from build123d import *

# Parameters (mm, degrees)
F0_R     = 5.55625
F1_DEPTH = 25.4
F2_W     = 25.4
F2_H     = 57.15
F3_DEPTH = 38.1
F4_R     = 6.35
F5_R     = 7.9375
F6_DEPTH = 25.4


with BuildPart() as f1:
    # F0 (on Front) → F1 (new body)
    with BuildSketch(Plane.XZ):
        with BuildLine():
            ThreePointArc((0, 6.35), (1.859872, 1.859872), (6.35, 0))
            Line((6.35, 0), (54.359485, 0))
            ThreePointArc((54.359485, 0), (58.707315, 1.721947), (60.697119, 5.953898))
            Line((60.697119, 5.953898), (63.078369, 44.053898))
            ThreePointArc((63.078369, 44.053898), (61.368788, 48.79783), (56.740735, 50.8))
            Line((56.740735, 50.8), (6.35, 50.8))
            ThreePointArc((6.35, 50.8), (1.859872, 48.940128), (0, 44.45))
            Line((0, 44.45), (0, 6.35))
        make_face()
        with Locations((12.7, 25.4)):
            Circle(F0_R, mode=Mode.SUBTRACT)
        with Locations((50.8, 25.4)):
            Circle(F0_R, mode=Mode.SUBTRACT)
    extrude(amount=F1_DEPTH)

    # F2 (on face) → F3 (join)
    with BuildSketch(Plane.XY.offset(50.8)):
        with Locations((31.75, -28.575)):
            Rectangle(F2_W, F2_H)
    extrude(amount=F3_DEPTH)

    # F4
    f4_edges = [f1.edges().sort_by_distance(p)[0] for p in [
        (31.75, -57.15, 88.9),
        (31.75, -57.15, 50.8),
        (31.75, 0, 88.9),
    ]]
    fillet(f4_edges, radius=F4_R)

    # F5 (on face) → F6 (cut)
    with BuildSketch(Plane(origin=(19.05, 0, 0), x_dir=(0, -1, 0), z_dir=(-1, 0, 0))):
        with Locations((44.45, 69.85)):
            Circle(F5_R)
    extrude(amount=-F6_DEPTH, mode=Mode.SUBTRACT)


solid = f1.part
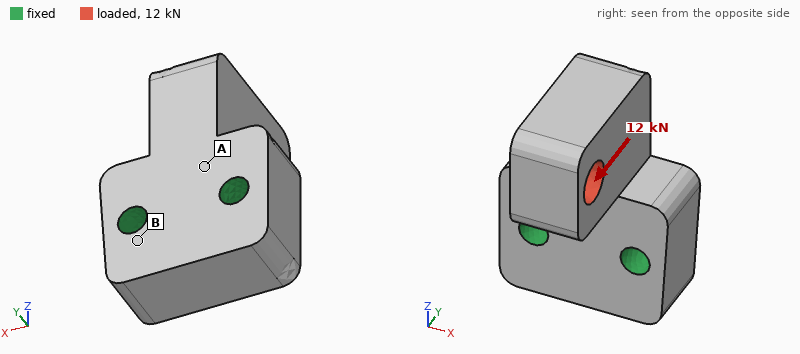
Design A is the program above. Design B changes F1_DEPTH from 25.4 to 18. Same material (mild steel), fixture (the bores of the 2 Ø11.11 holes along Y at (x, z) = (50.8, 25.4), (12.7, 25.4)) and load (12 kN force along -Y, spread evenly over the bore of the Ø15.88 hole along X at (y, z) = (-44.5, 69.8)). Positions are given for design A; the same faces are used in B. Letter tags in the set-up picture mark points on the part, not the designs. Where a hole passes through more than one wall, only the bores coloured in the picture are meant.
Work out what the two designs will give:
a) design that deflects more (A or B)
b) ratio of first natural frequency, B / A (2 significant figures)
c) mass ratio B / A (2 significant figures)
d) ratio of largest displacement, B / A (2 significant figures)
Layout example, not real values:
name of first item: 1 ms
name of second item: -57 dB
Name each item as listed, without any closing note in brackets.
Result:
design that deflects more: B
ratio of first natural frequency, B / A: 0.61
mass ratio B / A: 0.83
ratio of largest displacement, B / A: 2.5
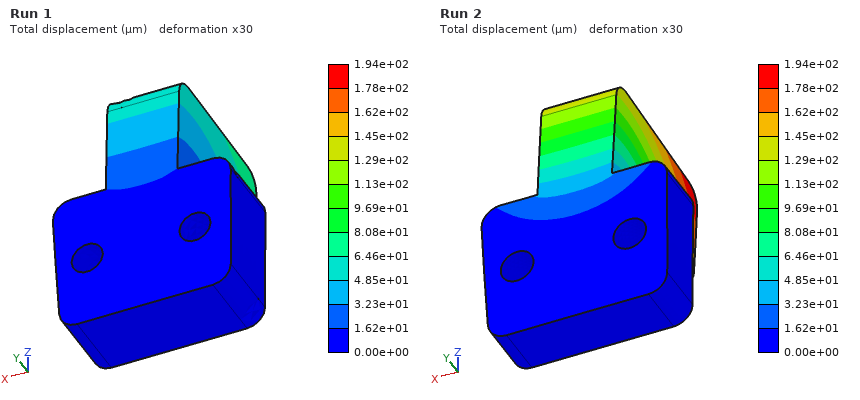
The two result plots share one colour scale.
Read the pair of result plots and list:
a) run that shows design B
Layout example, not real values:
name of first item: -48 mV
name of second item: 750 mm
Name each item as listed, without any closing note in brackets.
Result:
run that shows design B: Run 2
